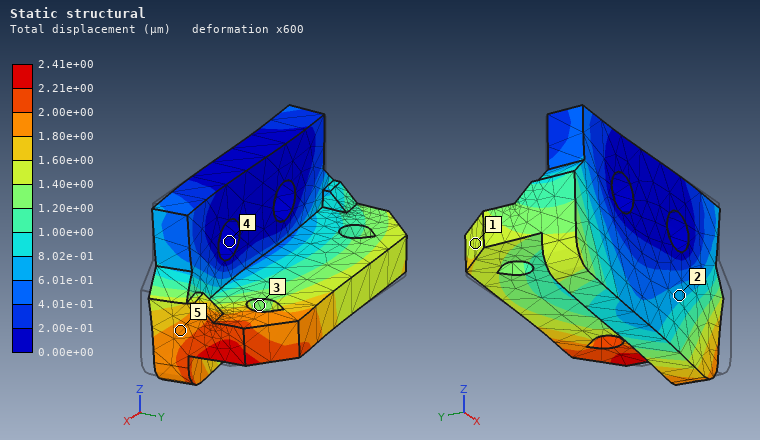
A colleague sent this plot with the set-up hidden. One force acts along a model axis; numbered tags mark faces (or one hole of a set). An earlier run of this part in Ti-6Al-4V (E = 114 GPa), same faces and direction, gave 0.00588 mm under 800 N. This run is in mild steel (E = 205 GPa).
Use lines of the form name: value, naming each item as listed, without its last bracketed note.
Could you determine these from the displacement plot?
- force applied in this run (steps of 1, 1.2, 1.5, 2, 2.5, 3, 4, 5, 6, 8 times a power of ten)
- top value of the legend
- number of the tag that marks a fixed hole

force applied in this run: 600 N
top value of the legend: 2.41e+00 µm
number of the tag that marks a fixed hole: 4
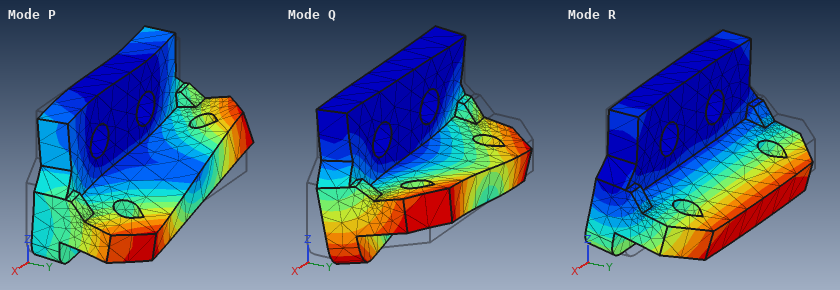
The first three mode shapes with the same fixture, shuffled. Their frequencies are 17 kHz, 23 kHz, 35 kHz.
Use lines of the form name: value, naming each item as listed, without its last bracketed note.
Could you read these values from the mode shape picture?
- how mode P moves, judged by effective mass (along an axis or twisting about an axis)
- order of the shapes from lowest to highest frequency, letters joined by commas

how mode P moves, judged by effective mass: along X
order of the shapes from lowest to highest frequency, letters joined by commas: R, Q, P
